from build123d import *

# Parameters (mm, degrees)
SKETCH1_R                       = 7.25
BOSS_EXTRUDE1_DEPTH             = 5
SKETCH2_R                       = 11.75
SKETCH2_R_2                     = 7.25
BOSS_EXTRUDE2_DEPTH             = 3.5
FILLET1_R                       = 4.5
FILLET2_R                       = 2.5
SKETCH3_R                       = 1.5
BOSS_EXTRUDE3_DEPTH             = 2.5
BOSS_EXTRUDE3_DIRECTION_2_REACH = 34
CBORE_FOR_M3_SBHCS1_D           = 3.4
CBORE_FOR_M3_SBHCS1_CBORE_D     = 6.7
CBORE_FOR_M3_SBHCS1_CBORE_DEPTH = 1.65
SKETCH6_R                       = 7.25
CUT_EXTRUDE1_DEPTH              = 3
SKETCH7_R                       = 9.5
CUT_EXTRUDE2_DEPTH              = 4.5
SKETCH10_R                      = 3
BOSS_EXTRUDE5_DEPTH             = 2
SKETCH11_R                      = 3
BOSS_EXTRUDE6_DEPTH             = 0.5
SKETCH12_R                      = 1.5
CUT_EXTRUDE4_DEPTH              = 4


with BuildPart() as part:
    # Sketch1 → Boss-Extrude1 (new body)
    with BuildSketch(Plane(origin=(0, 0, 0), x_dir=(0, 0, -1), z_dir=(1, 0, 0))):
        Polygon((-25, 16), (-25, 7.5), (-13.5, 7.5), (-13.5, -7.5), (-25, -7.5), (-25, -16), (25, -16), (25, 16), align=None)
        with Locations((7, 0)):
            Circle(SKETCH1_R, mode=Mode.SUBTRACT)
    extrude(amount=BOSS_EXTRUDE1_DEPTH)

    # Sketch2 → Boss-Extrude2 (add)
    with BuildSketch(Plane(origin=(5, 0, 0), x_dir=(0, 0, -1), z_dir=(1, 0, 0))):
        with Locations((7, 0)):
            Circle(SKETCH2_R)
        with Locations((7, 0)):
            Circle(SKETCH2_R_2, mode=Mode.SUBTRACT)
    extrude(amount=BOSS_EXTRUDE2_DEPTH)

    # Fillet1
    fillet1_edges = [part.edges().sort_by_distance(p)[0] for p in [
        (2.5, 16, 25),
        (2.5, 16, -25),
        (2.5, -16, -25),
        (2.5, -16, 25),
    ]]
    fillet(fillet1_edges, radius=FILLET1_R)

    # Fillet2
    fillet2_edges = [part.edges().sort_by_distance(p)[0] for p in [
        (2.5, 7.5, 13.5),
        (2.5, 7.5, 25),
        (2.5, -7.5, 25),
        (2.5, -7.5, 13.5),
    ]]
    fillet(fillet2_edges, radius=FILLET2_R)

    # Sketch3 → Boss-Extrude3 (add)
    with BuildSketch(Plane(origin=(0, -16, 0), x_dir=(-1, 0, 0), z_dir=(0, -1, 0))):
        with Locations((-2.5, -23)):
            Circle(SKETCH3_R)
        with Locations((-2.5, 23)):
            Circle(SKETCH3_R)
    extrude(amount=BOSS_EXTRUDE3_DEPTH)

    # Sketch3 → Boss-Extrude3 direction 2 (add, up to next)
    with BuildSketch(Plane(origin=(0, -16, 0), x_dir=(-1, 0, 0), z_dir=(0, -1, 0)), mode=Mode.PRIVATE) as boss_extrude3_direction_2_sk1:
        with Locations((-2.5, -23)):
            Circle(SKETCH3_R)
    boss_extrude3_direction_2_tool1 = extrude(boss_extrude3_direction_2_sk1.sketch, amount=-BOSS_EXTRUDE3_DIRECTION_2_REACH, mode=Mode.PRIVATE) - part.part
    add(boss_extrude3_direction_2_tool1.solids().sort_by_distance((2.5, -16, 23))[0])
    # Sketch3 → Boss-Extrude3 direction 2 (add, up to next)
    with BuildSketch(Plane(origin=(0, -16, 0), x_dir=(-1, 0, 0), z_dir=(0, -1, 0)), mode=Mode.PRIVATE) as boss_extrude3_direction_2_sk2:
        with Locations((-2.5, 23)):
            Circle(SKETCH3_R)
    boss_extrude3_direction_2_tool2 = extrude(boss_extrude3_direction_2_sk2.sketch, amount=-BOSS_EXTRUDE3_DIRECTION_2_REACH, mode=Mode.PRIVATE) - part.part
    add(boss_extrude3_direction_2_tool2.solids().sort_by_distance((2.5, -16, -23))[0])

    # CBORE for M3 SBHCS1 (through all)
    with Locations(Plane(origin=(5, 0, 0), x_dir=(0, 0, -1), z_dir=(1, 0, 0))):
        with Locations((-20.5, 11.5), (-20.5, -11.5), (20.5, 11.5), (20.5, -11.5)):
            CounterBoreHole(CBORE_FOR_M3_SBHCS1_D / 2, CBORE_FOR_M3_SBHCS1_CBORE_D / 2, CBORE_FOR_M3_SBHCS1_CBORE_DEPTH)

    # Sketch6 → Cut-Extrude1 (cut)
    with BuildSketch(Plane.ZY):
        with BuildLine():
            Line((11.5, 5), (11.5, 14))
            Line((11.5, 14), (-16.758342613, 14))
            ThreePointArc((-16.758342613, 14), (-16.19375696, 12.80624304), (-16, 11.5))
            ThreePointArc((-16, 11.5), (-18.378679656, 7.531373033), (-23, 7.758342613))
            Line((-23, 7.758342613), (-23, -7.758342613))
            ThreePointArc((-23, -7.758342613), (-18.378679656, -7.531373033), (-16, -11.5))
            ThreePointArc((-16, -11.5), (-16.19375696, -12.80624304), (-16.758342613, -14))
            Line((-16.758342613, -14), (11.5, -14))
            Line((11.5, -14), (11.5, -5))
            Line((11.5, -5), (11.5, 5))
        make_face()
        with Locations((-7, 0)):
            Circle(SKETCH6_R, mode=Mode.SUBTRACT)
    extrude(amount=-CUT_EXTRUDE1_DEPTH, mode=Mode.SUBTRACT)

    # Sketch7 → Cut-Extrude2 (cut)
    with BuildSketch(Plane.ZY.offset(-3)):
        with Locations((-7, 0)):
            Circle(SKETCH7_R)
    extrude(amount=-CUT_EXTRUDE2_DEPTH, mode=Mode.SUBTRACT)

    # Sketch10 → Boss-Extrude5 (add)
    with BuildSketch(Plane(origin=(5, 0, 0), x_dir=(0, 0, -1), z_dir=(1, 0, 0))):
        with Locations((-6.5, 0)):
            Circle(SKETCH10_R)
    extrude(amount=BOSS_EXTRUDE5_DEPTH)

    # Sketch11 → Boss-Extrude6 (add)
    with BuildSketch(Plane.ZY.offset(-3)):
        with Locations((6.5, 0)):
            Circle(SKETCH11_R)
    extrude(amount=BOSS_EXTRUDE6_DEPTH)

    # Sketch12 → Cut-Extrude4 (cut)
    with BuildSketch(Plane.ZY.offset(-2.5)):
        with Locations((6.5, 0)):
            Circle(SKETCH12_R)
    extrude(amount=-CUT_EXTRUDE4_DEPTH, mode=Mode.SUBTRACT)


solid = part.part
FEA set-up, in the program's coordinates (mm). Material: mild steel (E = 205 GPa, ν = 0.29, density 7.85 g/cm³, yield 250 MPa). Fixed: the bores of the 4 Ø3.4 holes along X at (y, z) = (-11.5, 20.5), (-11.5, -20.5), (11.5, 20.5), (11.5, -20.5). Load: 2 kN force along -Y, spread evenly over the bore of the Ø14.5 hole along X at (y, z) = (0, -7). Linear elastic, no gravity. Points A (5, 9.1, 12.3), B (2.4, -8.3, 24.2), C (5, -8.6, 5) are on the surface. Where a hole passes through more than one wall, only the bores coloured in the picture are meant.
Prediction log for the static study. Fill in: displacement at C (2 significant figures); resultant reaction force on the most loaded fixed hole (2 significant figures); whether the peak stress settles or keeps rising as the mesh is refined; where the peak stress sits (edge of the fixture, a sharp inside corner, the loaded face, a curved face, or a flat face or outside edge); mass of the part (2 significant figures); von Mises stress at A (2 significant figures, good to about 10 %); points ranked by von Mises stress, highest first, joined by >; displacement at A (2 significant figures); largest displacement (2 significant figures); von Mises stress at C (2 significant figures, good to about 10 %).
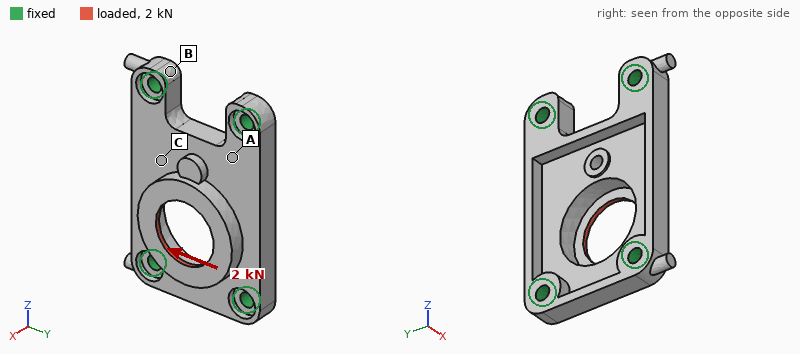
5.1 µm
760 N
keeps rising
edge of the fixture
33 g
17 MPa
C > A > B
2.9 µm
10 µm
34 MPa
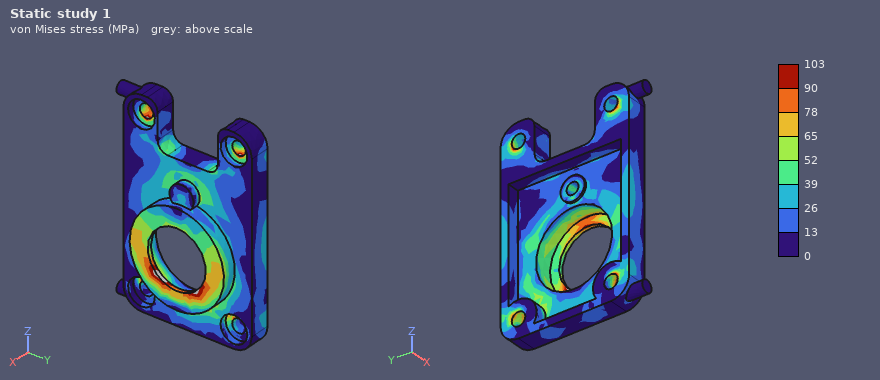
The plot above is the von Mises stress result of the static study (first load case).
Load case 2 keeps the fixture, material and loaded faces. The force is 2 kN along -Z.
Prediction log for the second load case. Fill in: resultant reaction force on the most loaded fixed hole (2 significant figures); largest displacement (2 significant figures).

530 N
9.3 µm
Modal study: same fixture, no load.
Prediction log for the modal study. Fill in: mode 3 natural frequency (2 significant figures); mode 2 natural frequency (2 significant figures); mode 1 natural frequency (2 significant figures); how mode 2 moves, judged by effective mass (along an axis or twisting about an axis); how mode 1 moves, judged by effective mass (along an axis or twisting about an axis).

21 kHz
15 kHz
12 kHz
twisting about Z
along X
